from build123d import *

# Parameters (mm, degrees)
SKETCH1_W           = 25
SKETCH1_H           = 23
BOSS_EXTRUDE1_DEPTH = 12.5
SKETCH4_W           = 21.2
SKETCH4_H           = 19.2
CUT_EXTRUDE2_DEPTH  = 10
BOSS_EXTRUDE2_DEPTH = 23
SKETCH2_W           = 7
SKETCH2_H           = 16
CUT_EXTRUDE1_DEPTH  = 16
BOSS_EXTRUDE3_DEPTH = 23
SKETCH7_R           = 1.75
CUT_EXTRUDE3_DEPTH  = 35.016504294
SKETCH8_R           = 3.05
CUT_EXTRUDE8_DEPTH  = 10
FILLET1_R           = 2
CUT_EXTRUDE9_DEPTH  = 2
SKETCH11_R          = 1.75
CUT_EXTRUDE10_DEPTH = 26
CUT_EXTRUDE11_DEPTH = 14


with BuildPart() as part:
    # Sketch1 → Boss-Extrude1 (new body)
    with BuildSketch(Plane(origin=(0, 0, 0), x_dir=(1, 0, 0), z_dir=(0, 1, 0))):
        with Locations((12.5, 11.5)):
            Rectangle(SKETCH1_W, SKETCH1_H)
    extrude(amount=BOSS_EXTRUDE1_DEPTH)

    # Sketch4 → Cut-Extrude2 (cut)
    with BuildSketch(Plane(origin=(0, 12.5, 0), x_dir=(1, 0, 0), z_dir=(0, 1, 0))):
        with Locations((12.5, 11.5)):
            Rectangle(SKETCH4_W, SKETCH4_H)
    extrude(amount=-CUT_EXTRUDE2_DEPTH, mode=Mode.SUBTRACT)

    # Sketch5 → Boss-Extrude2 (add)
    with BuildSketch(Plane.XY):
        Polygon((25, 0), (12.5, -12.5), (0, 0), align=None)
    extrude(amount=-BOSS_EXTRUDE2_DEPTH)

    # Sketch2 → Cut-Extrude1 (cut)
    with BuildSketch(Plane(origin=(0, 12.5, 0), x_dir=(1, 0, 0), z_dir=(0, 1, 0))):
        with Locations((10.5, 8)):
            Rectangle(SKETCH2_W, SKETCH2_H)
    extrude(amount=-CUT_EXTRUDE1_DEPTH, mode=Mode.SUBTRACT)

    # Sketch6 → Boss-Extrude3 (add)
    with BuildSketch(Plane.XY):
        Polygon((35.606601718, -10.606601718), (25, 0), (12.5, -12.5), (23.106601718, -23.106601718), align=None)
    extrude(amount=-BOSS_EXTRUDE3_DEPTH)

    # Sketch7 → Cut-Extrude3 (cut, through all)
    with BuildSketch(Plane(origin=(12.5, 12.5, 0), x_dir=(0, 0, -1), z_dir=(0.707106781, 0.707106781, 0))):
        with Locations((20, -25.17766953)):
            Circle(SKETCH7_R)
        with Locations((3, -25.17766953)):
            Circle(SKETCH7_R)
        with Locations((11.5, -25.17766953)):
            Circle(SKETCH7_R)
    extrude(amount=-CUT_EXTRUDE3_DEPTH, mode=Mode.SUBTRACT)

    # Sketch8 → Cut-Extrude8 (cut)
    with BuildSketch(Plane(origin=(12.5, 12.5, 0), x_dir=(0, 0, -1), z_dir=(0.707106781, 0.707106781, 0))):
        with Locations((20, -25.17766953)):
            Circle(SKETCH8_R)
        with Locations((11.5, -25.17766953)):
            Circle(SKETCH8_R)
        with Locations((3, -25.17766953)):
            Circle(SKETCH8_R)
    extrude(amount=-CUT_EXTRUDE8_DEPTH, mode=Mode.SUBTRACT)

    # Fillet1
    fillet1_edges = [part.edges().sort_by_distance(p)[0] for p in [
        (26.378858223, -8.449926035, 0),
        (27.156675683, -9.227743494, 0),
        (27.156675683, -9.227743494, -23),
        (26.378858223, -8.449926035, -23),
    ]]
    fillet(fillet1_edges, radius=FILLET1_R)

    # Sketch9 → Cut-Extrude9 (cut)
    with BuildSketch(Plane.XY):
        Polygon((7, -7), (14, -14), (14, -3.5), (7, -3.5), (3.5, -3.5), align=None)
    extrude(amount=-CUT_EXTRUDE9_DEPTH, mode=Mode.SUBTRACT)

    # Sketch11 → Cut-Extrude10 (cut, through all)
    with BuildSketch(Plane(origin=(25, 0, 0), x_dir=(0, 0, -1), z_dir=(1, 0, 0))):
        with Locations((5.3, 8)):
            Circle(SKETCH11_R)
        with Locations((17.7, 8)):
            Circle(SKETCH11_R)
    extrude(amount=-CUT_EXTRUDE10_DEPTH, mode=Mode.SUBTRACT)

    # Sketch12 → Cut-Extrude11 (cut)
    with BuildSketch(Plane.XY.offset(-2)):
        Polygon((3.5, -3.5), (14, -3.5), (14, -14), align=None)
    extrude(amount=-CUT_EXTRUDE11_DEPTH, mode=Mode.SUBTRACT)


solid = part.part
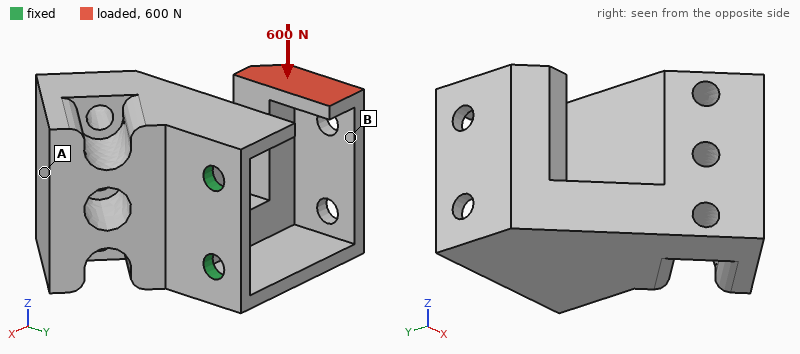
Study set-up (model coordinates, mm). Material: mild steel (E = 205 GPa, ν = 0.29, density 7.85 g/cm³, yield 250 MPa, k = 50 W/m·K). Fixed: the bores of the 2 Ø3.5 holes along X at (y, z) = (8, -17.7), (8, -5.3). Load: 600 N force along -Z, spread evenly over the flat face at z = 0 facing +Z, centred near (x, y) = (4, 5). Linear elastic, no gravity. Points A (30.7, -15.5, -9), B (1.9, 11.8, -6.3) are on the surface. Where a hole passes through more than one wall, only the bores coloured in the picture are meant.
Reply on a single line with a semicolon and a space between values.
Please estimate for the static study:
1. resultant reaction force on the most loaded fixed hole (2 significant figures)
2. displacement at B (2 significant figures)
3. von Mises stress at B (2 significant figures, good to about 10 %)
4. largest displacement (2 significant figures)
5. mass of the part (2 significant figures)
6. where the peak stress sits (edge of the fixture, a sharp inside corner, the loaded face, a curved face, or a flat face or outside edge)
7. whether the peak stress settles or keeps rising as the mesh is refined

770 N; 58 µm; 64 MPa; 68 µm; 77 g; edge of the fixture; keeps rising
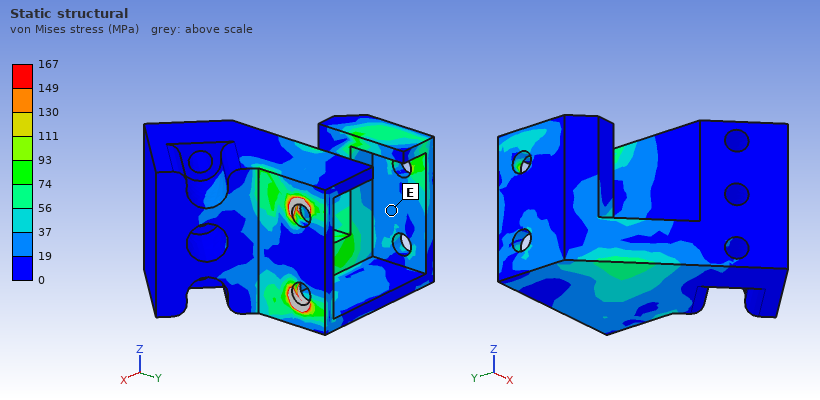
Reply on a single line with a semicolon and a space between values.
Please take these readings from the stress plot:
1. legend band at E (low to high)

19 to 37 MPa
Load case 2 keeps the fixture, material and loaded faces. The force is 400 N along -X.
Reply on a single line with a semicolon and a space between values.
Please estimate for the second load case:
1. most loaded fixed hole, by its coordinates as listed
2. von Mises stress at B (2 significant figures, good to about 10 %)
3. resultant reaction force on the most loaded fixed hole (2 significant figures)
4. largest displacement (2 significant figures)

(8, -5.3); 38 MPa; 470 N; 0.11 mm
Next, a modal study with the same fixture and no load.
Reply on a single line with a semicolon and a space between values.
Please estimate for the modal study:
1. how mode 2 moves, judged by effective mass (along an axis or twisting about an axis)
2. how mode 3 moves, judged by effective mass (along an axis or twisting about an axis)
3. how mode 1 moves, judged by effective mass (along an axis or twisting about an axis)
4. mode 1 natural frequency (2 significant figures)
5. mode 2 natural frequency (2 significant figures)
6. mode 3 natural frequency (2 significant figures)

along Z; along X; along X; 1500 Hz; 4500 Hz; 6400 Hz
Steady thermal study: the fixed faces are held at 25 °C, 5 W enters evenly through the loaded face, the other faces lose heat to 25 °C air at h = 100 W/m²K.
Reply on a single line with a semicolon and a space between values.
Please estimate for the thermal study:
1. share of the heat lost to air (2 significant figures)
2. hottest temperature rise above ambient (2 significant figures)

75 %; 45 K
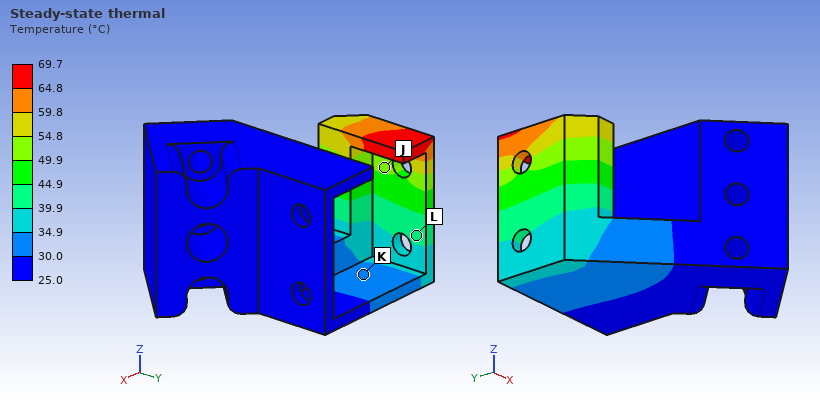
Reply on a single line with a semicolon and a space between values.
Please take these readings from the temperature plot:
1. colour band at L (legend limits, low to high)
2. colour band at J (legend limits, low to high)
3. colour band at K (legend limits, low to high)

39.9 to 44.9 °C; 49.9 to 54.8 °C; 30.0 to 34.9 °C
